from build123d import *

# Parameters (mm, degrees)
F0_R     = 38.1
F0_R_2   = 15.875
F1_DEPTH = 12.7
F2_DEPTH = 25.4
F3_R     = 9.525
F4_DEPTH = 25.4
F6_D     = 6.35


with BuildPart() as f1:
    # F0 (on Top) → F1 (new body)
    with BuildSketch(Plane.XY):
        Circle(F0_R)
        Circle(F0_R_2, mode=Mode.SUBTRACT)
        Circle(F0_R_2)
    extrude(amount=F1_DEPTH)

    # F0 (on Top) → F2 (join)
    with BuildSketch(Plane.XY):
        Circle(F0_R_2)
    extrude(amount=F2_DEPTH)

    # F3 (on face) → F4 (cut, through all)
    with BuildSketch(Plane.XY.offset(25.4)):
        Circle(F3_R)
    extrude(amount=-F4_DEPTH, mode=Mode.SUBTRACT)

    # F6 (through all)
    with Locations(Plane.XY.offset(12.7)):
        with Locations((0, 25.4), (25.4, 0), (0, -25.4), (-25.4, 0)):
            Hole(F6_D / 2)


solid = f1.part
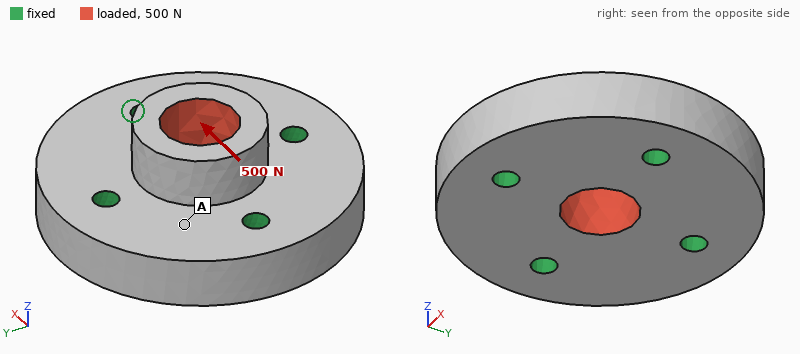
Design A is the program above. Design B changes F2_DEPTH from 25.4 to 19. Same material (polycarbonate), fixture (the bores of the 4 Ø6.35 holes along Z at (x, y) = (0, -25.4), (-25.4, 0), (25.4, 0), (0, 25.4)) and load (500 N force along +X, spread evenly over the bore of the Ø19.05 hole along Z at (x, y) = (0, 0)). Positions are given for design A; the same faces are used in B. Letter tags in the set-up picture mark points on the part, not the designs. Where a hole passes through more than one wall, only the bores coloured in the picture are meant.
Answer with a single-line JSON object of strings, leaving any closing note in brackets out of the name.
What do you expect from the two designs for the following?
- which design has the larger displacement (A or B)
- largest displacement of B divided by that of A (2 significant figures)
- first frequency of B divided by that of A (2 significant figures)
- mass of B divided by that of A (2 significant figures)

{"which design has the larger displacement": "A", "largest displacement of B divided by that of A": "0.55", "first frequency of B divided by that of A": "0.99", "mass of B divided by that of A": "0.95"}
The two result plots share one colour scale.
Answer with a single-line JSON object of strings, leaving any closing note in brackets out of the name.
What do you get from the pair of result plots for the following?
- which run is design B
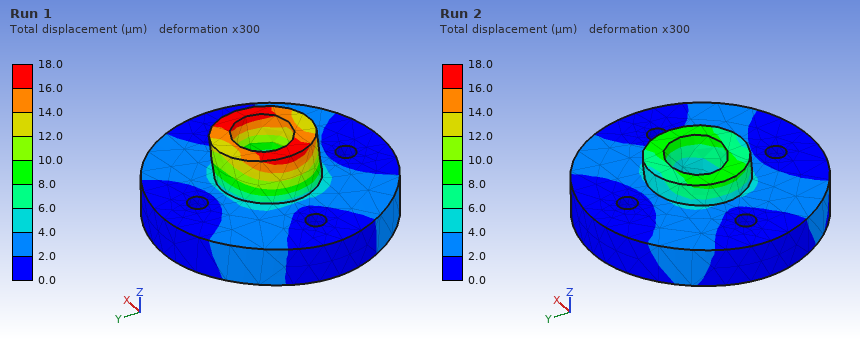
{"which run is design B": "Run 2"}
